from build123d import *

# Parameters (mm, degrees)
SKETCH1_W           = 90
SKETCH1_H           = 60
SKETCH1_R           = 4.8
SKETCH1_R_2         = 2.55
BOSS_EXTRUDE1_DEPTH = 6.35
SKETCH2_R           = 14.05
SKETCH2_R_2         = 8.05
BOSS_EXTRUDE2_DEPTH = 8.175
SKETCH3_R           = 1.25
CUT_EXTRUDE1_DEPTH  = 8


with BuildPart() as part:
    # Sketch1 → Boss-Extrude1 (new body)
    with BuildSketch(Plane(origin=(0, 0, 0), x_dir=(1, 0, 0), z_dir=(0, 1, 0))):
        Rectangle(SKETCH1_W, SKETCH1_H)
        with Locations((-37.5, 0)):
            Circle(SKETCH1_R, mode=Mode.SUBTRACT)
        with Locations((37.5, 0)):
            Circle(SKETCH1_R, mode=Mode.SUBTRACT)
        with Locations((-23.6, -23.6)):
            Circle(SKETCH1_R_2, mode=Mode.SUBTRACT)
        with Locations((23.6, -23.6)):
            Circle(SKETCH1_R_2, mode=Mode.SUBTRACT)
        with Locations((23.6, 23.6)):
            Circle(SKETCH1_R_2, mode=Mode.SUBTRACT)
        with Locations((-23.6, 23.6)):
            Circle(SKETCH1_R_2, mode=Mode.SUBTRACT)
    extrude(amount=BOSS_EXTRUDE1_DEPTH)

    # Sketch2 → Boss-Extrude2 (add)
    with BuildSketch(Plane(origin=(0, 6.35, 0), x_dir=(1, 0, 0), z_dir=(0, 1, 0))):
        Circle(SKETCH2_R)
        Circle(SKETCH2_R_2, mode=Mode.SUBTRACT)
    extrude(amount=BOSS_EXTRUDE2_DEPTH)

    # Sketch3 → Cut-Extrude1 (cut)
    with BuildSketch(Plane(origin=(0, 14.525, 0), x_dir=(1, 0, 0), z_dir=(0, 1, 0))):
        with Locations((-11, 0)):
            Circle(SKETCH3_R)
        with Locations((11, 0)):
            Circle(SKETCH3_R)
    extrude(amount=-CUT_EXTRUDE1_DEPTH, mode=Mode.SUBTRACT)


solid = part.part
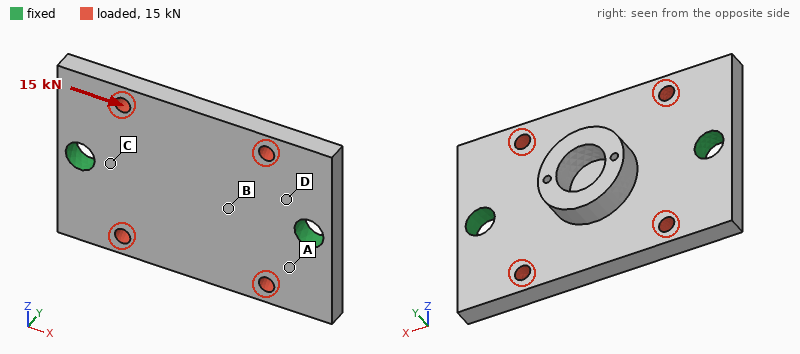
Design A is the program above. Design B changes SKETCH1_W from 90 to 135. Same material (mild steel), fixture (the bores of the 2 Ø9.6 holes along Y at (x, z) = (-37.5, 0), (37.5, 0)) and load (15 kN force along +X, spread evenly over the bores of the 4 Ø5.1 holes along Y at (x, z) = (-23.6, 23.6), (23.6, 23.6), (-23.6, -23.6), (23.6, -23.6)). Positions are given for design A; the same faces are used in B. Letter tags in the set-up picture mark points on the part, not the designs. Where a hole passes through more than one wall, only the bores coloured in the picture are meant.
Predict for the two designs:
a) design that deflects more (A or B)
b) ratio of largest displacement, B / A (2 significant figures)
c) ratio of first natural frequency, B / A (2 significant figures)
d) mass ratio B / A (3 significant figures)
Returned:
A
0.70
1.1
1.47
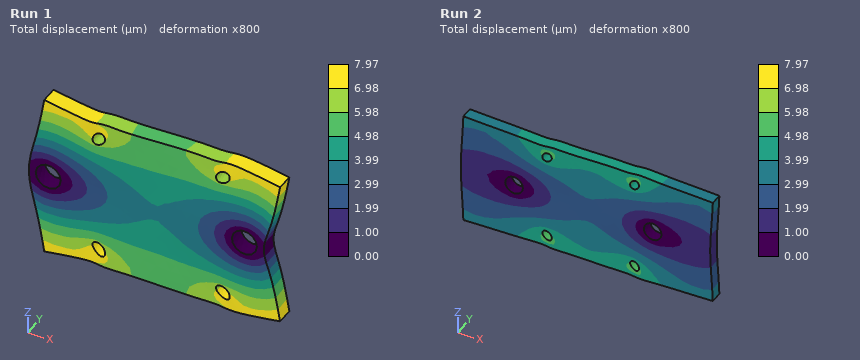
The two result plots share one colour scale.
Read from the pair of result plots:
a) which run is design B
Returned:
Run 2
